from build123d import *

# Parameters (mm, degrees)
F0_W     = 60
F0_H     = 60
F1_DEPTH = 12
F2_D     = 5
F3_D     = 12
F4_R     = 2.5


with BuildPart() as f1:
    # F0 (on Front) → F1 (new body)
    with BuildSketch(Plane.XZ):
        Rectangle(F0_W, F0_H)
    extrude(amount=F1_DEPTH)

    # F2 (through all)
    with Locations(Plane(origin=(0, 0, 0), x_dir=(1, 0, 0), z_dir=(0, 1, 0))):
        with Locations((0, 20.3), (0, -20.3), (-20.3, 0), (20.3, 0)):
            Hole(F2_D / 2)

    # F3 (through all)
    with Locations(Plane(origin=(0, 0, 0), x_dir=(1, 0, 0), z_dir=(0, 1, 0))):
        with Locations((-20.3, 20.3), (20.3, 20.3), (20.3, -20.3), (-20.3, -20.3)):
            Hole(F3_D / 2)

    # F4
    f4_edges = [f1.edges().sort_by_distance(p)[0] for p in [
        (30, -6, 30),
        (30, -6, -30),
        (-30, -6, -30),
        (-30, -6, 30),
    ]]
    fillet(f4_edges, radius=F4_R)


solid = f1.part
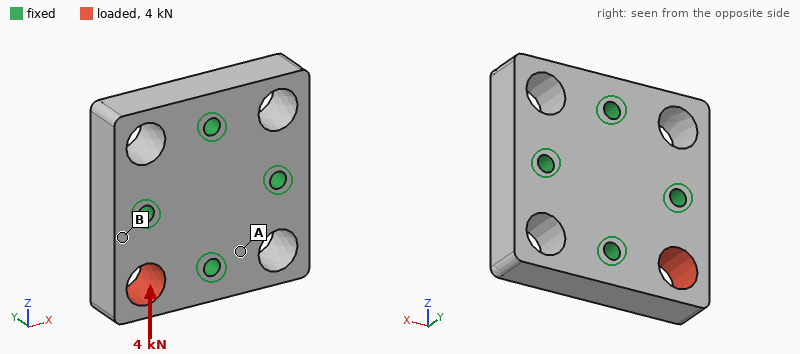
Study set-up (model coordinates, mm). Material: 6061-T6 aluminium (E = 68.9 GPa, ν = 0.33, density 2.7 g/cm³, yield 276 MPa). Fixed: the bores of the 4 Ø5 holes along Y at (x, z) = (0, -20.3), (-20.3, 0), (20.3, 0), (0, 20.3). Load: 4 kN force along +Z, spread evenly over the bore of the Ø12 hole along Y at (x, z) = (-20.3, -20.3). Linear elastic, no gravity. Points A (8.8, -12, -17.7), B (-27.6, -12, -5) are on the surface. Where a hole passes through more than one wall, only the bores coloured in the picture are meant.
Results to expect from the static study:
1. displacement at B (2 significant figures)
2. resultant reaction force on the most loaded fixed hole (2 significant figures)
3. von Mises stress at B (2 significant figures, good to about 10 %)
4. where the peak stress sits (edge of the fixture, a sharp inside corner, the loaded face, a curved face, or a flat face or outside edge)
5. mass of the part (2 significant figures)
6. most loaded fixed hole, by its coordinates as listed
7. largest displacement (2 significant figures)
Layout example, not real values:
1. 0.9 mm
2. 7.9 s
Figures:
1. 2.8 µm
2. 2.9 kN
3. 15 MPa
4. the loaded face
5. 99 g
6. (-20.3, 0)
7. 12 µm
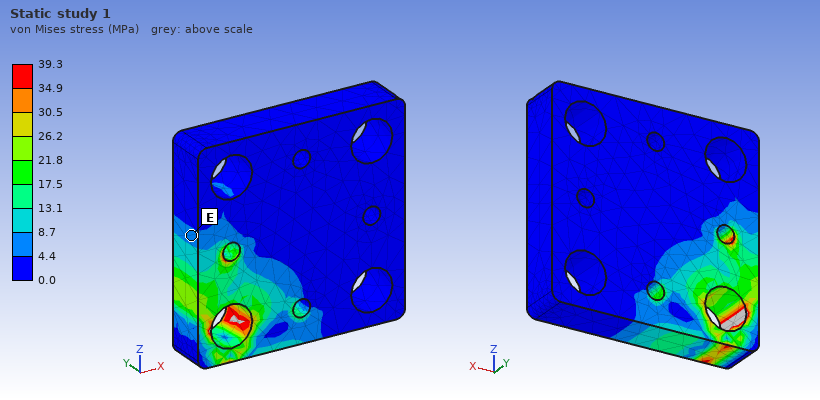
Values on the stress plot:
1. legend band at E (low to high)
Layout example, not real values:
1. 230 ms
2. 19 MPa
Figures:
1. 4.4 to 8.7 MPa
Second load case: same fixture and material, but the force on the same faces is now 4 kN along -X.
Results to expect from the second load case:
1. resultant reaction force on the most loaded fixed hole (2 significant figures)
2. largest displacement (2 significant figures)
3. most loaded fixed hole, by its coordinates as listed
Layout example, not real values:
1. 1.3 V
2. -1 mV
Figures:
1. 2.9 kN
2. 12 µm
3. (0, -20.3)
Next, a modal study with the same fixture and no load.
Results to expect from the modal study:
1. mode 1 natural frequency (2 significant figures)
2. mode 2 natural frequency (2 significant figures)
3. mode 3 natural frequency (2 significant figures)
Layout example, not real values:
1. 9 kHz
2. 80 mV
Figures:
1. 17 kHz
2. 17 kHz
3. 17 kHz
